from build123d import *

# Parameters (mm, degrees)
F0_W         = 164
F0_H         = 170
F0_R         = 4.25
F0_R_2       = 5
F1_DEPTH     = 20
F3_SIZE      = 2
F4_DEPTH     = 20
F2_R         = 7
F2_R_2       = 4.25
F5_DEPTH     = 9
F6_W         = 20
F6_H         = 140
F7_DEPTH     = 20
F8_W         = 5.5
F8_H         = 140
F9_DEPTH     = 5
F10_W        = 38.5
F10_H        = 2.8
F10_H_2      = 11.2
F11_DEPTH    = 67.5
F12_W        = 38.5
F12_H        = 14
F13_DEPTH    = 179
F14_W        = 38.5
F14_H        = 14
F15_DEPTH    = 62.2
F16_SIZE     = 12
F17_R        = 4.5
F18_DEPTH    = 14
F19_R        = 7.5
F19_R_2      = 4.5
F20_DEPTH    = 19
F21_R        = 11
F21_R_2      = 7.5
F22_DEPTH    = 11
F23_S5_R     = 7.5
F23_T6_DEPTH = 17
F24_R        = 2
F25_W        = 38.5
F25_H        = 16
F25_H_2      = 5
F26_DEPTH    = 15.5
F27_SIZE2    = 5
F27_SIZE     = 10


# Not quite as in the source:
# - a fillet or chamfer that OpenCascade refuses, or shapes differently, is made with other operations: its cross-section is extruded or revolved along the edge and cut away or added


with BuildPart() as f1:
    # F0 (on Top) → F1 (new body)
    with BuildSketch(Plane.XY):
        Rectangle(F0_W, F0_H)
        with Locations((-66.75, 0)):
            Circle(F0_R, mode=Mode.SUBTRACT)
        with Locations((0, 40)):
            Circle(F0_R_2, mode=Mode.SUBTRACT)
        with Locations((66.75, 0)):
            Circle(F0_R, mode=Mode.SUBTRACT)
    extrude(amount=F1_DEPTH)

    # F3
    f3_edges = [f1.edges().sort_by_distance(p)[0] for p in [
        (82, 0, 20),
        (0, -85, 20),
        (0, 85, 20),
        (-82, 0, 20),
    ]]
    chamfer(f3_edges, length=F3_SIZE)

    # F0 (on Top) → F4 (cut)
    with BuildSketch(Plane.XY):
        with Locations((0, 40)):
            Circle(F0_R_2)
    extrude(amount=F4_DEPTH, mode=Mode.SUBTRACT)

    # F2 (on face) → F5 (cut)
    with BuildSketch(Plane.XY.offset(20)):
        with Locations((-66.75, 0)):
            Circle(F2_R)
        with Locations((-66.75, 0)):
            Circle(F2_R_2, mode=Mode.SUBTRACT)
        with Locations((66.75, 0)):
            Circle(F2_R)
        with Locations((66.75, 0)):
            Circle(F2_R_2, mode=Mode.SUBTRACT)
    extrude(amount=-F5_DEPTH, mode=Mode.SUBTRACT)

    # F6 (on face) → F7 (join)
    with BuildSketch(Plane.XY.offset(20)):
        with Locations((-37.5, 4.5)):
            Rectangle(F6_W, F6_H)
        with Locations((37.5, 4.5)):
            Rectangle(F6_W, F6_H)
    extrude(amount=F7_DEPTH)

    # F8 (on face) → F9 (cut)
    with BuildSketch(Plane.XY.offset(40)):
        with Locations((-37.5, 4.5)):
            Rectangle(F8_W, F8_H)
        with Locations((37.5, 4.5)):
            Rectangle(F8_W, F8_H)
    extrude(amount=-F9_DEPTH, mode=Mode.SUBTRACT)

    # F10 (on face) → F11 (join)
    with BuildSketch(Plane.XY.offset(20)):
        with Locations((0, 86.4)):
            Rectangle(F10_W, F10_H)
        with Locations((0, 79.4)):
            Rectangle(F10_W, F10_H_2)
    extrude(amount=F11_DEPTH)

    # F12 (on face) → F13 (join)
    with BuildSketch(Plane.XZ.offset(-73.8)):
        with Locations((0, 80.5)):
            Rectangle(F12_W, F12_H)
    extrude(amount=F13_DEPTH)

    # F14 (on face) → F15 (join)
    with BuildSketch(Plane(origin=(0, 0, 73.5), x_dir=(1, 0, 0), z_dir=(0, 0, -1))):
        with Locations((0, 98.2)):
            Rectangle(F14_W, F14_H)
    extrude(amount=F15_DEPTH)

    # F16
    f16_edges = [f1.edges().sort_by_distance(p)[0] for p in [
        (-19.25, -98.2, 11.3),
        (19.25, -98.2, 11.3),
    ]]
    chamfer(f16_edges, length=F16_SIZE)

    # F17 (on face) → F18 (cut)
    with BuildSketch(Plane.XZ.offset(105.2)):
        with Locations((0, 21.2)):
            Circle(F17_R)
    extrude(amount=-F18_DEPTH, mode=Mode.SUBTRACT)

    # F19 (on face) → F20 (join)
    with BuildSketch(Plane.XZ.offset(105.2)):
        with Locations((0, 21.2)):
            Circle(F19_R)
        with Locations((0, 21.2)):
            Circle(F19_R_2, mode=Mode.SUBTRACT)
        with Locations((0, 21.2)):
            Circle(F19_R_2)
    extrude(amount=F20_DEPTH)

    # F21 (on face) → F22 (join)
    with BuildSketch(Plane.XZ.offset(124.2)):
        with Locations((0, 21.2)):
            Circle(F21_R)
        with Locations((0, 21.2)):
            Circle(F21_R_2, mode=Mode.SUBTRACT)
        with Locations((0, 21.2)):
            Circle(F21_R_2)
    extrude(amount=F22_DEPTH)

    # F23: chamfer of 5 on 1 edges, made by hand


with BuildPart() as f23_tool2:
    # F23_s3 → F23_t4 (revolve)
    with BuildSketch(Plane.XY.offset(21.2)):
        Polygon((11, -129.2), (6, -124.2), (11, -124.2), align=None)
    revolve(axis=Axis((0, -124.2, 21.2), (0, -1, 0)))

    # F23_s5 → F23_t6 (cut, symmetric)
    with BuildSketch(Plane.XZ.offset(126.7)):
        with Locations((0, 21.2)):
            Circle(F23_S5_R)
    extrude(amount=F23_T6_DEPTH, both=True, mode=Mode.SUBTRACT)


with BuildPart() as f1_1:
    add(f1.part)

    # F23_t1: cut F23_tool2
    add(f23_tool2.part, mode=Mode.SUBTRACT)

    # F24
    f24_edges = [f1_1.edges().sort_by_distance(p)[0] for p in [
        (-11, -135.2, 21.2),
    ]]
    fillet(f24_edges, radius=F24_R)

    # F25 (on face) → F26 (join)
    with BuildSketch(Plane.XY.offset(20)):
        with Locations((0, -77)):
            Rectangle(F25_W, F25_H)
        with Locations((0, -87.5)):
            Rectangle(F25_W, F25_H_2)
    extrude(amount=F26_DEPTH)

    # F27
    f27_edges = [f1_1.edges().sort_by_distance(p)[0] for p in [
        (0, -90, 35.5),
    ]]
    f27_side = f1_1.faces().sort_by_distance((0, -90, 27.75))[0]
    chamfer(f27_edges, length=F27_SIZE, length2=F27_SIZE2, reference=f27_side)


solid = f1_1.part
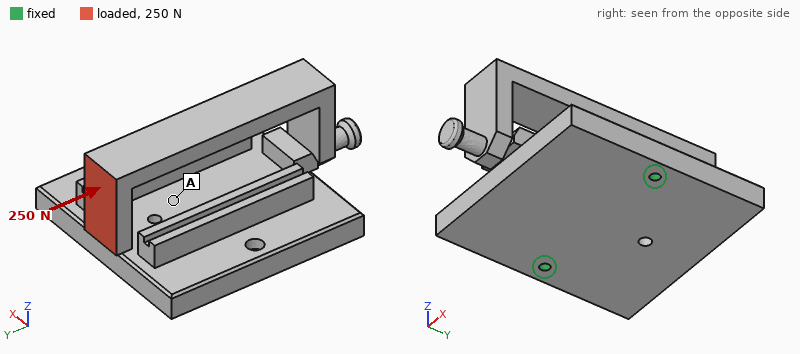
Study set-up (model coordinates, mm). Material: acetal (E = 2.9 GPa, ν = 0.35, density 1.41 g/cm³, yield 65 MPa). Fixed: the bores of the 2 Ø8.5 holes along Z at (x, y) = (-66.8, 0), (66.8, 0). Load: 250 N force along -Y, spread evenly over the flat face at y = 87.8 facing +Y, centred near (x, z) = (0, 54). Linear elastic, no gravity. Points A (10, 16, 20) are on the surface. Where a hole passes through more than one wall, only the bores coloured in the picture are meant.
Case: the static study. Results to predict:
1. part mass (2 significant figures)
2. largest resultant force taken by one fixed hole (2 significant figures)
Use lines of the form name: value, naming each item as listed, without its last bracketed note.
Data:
part mass: 1.2 kg
largest resultant force taken by one fixed hole: 130 N
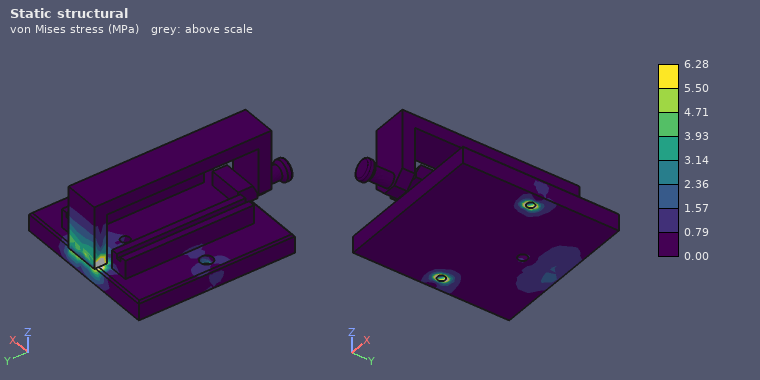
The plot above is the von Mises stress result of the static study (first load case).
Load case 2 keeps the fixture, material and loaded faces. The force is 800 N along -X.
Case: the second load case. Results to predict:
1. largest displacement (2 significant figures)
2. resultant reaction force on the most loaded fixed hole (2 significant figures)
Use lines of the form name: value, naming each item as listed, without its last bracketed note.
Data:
largest displacement: 0.89 mm
resultant reaction force on the most loaded fixed hole: 720 N
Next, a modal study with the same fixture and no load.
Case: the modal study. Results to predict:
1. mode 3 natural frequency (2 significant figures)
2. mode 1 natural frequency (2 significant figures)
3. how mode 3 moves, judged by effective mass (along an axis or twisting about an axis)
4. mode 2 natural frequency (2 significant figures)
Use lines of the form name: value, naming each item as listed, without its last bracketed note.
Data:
mode 3 natural frequency: 140 Hz
mode 1 natural frequency: 38 Hz
how mode 3 moves, judged by effective mass: along Y
mode 2 natural frequency: 56 Hz
